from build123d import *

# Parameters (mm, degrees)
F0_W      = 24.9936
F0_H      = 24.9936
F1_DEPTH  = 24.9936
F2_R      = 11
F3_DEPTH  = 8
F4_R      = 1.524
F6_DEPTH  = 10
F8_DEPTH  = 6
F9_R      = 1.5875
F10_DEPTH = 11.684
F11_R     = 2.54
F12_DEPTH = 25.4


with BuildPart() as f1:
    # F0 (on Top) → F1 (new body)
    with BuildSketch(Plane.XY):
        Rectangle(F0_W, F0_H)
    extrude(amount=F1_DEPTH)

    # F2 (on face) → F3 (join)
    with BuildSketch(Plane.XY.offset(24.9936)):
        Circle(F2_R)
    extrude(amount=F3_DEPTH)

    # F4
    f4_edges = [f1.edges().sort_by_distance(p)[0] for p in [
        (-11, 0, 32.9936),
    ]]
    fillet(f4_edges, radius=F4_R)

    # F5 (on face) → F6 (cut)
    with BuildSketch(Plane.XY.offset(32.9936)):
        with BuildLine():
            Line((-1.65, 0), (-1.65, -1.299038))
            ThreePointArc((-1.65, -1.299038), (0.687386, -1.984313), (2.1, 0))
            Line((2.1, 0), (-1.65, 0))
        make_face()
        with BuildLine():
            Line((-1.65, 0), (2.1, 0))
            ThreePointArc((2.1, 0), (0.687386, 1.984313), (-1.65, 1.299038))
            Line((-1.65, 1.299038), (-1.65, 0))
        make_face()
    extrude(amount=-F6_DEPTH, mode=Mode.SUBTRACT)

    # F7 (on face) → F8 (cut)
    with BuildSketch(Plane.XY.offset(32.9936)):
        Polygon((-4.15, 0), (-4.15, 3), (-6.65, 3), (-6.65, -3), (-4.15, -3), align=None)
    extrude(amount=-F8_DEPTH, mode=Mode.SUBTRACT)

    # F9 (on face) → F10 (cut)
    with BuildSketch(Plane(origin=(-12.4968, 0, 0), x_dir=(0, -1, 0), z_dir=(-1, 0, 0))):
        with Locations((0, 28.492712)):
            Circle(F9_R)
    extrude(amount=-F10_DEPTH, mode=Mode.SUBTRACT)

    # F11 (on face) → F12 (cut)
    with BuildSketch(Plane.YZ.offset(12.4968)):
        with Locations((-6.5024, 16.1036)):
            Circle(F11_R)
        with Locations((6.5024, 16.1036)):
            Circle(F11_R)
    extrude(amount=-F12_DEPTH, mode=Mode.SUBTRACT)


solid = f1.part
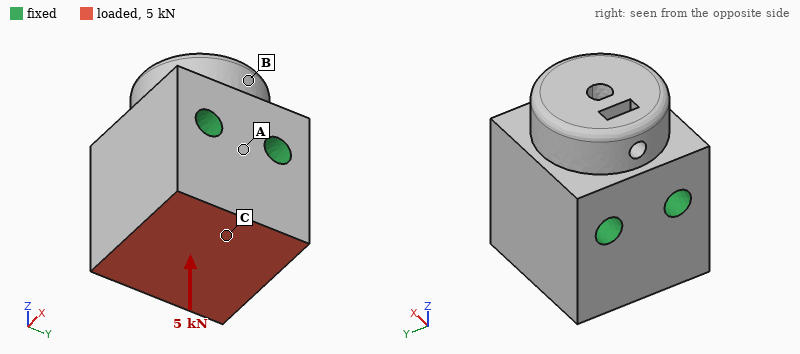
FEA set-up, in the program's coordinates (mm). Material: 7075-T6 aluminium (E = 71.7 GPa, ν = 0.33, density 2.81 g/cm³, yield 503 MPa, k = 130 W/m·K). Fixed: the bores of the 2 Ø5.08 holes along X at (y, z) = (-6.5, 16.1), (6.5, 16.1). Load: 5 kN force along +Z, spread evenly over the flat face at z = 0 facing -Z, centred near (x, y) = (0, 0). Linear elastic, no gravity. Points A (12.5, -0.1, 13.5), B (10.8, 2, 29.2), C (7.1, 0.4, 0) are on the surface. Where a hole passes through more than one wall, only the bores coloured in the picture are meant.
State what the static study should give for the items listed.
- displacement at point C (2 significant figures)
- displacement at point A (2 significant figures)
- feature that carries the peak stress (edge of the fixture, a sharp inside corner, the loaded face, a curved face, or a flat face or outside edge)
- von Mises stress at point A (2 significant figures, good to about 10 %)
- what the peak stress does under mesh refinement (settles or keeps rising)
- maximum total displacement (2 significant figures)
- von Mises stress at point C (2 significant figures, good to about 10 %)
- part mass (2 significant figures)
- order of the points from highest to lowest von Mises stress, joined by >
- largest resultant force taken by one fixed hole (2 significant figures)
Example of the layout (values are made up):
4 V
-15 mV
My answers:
1.7 µm
0.53 µm
edge of the fixture
3.7 MPa
keeps rising
2.0 µm
8.6 MPa
49 g
C > A > B
2.5 kN
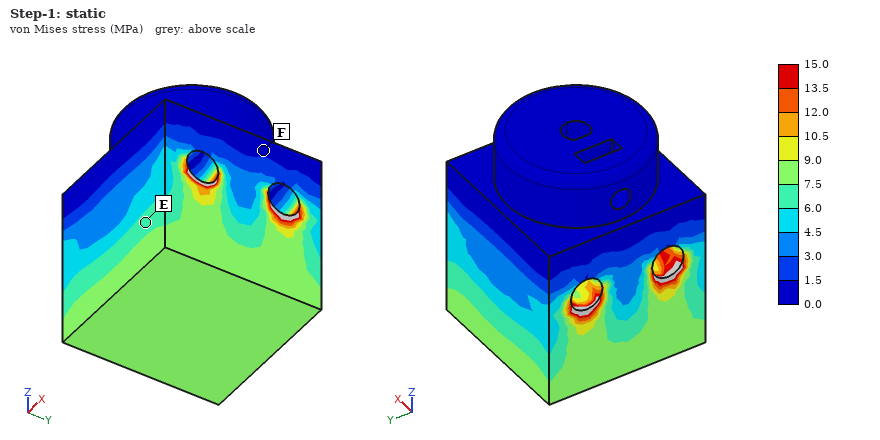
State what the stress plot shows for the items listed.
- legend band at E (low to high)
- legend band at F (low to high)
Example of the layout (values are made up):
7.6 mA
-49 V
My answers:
6.0 to 7.5 MPa
0.0 to 1.5 MPa
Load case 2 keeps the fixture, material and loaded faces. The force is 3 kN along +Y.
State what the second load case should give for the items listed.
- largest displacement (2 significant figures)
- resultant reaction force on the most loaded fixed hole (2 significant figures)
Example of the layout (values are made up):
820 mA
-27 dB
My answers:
6.3 µm
3.1 kN
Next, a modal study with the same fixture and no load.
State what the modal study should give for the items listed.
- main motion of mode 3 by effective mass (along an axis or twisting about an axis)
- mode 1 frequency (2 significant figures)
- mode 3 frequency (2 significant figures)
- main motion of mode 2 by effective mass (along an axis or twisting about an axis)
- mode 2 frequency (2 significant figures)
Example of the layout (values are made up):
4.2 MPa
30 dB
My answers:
along Y
39 kHz
45 kHz
along X
41 kHz
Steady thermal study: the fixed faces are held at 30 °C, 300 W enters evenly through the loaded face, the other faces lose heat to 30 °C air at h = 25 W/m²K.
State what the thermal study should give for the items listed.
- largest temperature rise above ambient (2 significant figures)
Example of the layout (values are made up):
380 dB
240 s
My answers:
55 K
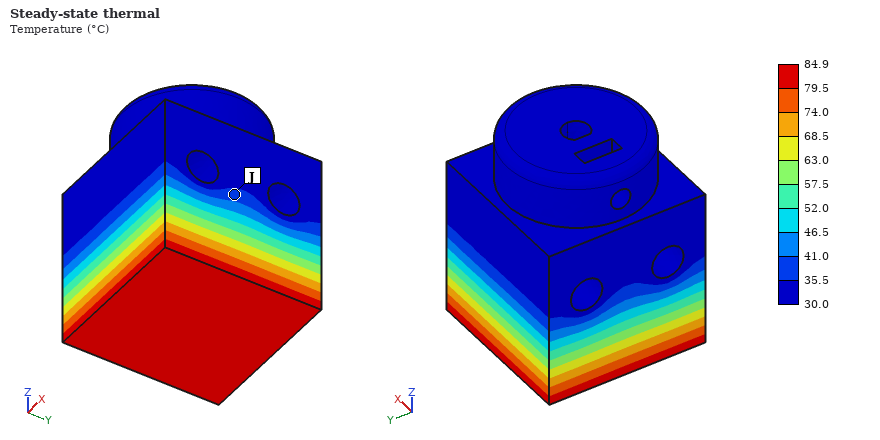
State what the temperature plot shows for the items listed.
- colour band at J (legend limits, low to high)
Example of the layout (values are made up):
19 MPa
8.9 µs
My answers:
35.5 to 41.0 °C
